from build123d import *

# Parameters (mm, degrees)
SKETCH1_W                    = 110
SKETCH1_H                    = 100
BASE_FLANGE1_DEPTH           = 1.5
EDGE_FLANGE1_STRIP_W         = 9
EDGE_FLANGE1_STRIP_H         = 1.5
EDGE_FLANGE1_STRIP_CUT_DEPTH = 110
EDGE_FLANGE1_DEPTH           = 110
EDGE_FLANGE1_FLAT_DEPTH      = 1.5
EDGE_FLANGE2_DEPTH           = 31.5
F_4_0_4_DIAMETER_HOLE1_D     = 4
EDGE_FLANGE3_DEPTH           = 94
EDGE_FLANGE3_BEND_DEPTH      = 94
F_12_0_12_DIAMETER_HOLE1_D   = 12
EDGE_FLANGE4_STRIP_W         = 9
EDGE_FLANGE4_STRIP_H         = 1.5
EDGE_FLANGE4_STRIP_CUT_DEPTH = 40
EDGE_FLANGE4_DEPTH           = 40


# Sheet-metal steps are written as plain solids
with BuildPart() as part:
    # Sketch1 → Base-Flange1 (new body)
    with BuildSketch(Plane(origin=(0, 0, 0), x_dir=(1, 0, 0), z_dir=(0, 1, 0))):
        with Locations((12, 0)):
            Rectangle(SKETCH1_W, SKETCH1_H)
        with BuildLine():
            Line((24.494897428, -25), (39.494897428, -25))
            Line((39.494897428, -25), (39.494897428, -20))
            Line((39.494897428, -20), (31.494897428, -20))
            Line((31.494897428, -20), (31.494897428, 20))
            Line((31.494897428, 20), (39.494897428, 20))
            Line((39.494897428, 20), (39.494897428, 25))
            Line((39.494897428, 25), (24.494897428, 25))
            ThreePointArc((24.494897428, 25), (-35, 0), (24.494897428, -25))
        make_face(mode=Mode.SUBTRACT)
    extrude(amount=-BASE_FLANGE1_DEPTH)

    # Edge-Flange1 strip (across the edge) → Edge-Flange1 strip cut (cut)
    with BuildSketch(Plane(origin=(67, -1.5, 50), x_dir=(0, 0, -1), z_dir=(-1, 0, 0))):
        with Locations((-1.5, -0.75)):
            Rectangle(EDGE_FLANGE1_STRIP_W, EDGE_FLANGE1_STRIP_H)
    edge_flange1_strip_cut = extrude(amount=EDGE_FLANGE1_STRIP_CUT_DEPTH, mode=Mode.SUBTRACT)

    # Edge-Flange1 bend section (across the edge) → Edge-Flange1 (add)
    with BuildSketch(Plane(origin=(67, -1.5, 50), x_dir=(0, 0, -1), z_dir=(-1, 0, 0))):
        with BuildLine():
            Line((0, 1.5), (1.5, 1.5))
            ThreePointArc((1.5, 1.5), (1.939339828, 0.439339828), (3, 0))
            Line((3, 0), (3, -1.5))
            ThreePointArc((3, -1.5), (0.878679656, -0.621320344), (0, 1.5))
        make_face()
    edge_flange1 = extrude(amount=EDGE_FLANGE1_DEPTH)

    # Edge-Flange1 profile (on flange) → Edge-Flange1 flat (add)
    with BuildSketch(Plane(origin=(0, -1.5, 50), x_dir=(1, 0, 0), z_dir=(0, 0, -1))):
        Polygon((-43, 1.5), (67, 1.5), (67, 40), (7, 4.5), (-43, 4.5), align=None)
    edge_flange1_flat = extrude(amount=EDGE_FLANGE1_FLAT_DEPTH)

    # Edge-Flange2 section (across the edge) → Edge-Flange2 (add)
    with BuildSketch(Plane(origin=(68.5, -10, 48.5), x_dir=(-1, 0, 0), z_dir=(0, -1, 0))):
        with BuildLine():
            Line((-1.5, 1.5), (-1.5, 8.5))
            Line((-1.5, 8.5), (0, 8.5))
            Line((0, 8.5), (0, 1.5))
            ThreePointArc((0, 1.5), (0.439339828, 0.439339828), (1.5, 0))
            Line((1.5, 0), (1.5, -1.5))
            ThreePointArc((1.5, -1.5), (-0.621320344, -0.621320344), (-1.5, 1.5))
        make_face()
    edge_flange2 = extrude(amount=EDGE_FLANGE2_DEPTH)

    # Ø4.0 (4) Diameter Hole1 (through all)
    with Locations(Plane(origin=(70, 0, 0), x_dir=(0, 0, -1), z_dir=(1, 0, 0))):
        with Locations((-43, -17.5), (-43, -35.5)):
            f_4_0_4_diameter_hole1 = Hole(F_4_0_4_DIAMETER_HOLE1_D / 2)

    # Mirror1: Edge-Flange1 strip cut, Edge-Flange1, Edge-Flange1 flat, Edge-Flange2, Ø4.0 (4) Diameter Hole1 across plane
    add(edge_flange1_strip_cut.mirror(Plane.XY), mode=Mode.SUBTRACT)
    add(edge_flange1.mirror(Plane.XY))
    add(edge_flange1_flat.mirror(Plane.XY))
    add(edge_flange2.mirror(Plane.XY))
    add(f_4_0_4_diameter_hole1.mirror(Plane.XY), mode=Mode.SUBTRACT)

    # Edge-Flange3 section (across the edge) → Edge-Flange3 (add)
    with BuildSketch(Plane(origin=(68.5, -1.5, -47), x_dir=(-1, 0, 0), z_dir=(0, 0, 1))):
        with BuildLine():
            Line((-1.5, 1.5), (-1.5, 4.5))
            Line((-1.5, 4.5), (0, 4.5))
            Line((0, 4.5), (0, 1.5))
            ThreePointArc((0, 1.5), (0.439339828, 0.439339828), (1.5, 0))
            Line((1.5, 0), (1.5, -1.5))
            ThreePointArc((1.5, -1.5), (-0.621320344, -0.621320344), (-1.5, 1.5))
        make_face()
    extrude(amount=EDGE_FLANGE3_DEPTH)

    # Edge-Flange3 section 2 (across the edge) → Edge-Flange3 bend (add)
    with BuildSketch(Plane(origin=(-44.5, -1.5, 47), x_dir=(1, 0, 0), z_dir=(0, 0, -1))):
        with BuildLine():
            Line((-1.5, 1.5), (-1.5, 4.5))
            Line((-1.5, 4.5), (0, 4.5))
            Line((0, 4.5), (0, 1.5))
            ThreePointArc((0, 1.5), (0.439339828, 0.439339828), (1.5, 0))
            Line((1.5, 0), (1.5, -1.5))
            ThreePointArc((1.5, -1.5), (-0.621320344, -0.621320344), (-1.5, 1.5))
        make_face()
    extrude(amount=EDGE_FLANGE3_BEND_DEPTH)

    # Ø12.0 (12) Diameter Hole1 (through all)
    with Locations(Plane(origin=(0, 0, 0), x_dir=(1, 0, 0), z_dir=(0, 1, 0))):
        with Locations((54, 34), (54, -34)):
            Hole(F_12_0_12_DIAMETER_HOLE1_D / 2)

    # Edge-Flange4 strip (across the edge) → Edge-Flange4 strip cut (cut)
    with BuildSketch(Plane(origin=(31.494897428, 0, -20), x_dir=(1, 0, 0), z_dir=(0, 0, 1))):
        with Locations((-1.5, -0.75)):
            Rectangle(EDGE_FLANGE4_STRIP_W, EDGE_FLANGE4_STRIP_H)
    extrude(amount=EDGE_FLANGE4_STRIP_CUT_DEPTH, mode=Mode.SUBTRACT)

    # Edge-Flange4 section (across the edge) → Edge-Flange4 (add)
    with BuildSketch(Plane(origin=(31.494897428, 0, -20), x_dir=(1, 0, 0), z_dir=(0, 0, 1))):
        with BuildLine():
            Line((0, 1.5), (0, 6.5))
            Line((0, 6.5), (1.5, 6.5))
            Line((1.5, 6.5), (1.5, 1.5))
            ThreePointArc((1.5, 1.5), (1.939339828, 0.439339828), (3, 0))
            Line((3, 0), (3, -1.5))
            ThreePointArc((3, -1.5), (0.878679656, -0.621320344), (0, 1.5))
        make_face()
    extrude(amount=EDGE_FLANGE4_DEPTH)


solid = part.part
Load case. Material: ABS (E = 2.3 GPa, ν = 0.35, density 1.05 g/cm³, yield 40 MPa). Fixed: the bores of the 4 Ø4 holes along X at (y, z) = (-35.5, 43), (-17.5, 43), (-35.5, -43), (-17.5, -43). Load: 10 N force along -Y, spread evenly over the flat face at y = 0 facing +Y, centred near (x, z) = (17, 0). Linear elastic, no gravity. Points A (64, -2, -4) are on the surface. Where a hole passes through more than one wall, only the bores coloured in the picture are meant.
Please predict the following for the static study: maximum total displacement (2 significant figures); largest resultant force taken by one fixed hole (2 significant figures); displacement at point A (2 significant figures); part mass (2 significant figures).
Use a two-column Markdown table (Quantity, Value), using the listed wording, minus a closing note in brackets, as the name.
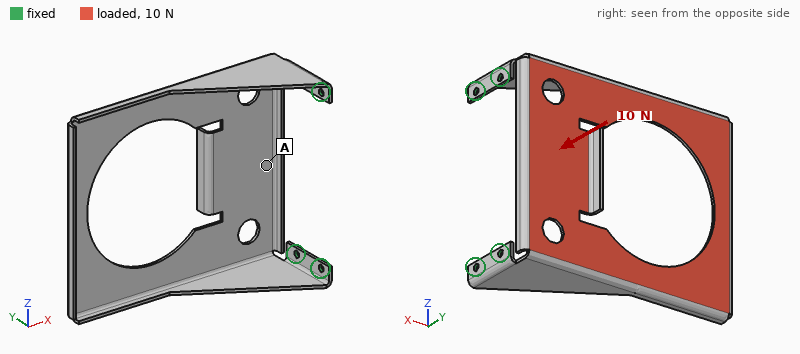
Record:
| Quantity | Value |
|---|---|
| maximum total displacement | 1.7 mm |
| largest resultant force taken by one fixed hole | 14 N |
| displacement at point A | 0.35 mm |
| part mass | 19 g |
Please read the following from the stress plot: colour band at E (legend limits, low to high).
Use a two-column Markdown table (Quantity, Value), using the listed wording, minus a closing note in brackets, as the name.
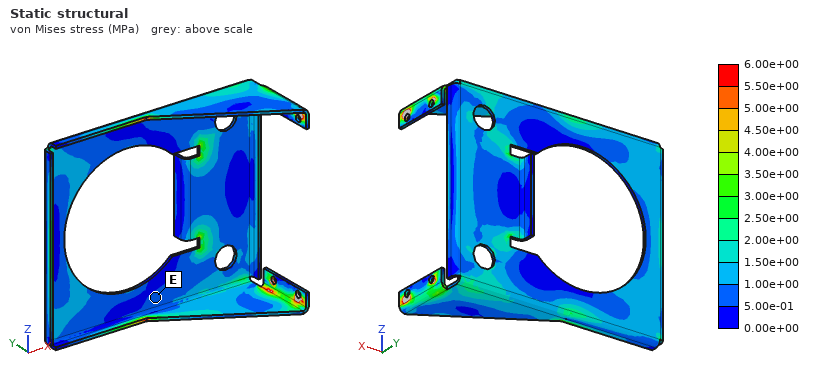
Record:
| Quantity | Value |
|---|---|
| colour band at E | 5.00e-01 to 1.00e+00 MPa |
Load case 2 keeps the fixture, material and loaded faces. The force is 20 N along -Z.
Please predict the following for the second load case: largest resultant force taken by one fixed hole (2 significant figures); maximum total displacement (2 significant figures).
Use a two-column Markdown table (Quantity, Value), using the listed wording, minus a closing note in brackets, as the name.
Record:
| Quantity | Value |
|---|---|
| largest resultant force taken by one fixed hole | 21 N |
| maximum total displacement | 1.6 mm |
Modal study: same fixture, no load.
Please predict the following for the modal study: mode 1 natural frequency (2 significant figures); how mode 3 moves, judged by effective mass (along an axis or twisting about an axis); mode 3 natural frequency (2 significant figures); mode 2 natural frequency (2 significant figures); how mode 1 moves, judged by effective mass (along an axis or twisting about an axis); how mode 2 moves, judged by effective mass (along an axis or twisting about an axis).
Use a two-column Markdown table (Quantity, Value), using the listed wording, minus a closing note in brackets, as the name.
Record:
| Quantity | Value |
|---|---|
| mode 1 natural frequency | 120 Hz |
| how mode 3 moves, judged by effective mass | along Y |
| mode 3 natural frequency | 230 Hz |
| mode 2 natural frequency | 150 Hz |
| how mode 1 moves, judged by effective mass | along Y |
| how mode 2 moves, judged by effective mass | along Z |
